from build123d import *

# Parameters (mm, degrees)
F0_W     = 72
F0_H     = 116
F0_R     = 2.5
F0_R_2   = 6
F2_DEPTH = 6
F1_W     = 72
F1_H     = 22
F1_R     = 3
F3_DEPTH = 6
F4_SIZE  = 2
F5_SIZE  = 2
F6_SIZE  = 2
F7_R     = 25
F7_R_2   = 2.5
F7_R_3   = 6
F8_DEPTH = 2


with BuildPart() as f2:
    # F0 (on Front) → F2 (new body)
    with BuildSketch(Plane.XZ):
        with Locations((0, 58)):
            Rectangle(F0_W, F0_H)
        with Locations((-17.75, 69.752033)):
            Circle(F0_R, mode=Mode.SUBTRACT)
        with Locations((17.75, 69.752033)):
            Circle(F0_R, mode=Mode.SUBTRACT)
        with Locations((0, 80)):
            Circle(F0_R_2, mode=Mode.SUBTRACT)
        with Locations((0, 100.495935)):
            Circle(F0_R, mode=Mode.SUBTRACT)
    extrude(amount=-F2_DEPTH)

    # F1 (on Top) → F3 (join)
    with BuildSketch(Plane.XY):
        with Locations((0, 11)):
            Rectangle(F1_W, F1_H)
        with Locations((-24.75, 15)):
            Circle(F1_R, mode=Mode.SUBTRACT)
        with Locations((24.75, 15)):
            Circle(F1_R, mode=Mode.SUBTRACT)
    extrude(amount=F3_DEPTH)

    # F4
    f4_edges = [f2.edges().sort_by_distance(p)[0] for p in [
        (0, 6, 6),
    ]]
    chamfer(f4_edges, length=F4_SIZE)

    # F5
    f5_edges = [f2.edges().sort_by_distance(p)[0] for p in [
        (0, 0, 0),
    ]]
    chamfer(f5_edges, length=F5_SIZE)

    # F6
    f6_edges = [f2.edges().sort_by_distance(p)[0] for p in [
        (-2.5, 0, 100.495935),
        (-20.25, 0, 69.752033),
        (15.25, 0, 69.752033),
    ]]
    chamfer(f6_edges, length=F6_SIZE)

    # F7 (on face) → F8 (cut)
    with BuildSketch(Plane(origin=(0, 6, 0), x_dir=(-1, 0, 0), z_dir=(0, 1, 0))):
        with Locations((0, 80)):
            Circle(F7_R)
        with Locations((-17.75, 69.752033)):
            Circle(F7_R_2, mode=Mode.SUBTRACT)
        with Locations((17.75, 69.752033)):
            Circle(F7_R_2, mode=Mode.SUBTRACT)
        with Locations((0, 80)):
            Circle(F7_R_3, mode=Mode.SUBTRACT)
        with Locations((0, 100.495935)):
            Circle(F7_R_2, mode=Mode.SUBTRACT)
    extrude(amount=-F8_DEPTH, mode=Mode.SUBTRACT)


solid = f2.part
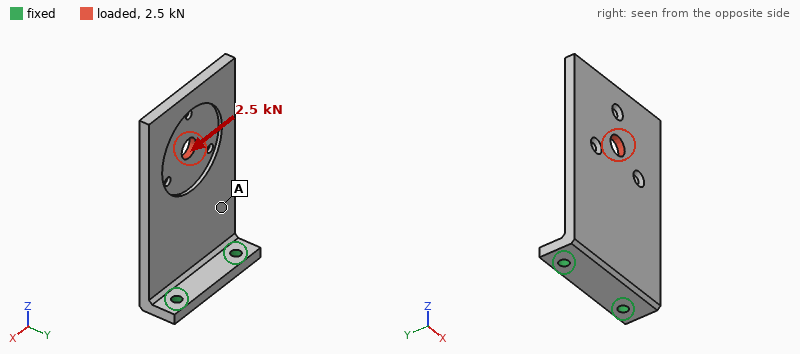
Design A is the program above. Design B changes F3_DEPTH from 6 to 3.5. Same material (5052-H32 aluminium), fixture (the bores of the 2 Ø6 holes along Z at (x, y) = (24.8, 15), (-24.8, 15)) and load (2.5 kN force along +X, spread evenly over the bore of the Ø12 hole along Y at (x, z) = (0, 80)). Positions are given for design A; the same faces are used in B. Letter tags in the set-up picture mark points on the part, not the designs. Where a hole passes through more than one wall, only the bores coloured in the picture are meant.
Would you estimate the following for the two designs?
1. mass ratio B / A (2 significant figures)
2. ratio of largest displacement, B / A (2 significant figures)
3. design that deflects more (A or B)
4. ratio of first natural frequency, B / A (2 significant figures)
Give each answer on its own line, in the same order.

0.95
2.1
B
0.69
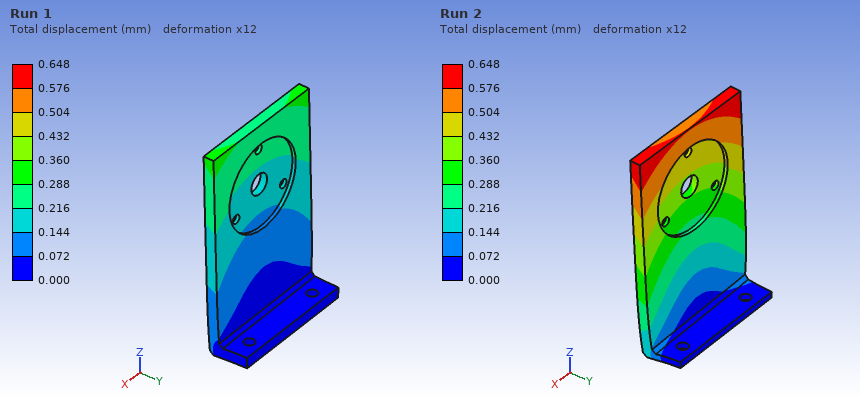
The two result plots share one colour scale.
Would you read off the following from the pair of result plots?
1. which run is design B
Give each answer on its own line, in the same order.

Run 2
